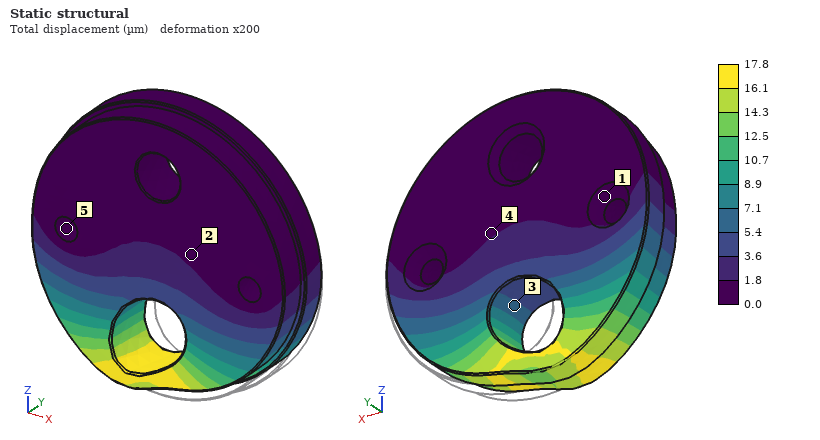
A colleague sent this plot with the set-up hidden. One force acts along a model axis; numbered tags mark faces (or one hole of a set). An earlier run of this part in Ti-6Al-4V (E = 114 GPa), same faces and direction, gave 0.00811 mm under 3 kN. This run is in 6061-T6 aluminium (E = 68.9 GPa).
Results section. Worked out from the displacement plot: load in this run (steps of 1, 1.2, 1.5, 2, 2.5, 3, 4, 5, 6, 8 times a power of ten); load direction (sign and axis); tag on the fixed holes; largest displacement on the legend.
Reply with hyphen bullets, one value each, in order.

- 4 kN
- -X
- 5
- 17.8 µm
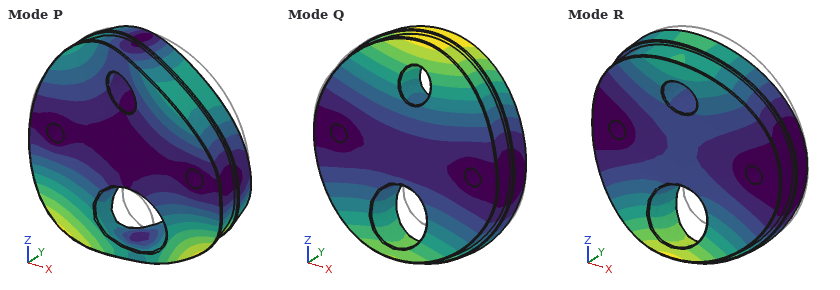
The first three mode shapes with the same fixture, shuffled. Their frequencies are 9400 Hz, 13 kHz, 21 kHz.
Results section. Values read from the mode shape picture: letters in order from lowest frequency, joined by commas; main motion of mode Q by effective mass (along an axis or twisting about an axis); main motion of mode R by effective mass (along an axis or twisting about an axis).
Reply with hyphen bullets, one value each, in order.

- Q, R, P
- twisting about X
- along Y
